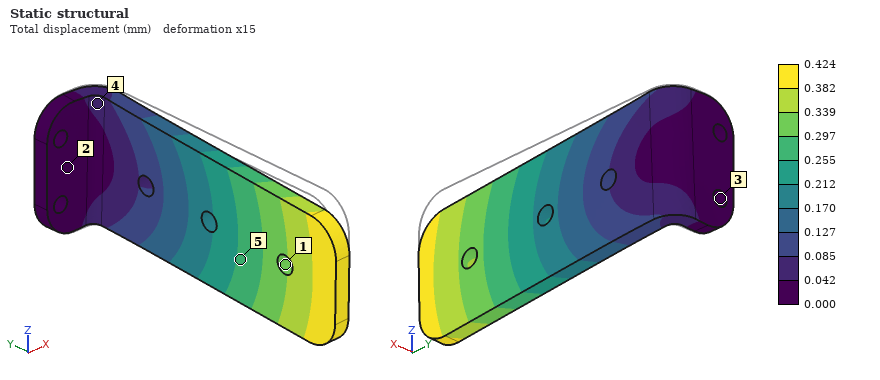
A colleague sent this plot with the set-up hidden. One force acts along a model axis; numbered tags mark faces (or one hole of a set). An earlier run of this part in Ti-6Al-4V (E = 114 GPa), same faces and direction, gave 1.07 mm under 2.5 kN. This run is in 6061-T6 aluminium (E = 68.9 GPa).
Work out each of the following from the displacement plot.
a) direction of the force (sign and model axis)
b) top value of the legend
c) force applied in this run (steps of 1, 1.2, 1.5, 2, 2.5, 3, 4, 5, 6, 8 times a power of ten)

-Z
0.424 mm
600 N
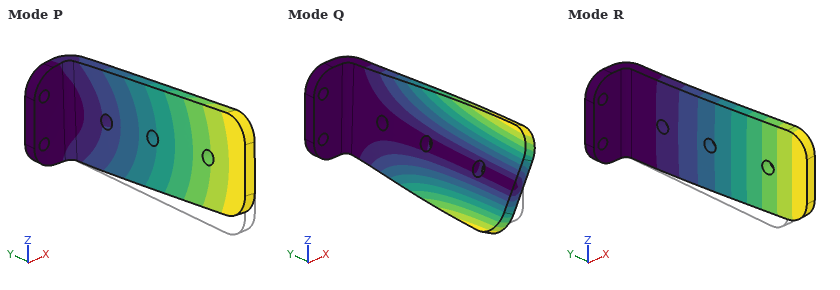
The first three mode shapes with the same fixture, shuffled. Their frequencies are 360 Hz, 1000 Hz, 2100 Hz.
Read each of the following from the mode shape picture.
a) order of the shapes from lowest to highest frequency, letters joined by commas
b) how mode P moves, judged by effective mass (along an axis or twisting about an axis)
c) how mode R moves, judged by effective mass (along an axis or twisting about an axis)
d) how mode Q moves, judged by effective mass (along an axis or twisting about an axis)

R, P, Q
along Z
along X
twisting about Y
